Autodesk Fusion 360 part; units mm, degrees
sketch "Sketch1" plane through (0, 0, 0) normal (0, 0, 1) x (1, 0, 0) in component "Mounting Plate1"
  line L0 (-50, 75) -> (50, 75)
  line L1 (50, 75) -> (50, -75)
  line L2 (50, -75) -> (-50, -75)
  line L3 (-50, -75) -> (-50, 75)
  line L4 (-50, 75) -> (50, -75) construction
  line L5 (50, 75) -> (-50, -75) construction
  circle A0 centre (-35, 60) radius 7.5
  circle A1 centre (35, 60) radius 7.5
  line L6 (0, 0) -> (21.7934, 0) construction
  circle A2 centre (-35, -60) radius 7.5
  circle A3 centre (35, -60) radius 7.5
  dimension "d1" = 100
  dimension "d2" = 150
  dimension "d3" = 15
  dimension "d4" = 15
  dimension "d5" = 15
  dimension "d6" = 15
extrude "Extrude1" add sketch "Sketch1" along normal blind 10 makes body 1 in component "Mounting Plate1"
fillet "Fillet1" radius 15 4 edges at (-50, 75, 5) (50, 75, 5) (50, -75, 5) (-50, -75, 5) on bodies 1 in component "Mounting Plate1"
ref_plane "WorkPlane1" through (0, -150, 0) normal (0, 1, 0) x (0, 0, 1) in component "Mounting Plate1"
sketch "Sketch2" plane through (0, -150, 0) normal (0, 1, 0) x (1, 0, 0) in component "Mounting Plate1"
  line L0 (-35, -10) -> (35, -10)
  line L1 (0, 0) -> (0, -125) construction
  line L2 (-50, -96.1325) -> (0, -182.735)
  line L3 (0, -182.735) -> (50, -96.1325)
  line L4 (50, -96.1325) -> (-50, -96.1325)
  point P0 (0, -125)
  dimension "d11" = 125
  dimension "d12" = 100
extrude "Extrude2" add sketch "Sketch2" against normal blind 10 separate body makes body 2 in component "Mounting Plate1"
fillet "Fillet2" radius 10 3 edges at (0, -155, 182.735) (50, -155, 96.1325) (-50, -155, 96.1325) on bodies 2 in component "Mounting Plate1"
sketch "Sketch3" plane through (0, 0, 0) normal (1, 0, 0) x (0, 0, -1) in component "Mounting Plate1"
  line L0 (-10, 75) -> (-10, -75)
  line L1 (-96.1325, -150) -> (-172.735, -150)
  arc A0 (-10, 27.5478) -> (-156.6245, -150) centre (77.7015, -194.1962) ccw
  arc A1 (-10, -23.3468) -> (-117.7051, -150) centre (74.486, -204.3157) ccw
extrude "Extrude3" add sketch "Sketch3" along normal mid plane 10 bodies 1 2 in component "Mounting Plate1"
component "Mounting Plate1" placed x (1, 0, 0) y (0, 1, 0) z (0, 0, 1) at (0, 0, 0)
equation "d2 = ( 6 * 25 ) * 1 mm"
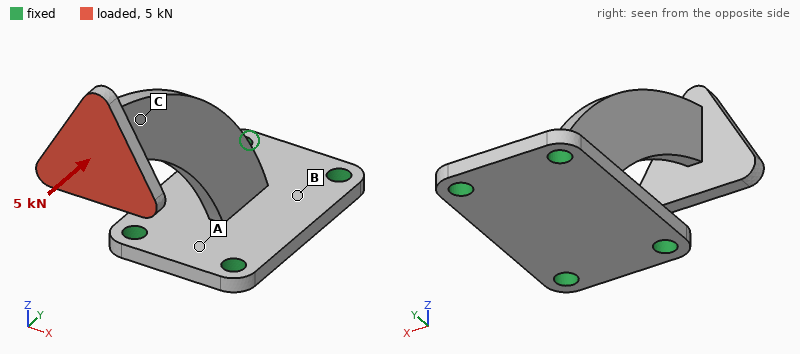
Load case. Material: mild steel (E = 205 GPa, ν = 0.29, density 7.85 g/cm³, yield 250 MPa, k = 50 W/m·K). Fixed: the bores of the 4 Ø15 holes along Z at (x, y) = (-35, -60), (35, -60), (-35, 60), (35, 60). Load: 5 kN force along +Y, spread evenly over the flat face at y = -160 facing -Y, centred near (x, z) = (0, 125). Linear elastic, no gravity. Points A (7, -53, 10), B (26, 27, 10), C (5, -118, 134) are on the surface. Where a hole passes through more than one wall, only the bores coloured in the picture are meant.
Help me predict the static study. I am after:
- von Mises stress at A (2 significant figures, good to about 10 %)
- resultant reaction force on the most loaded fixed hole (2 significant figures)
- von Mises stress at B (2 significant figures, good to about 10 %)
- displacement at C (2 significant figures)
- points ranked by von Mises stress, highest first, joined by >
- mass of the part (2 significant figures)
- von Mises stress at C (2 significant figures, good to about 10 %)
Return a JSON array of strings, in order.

["35 MPa", "3.9 kN", "49 MPa", "0.61 mm", "B > A > C", "2.1 kg", "14 MPa"]
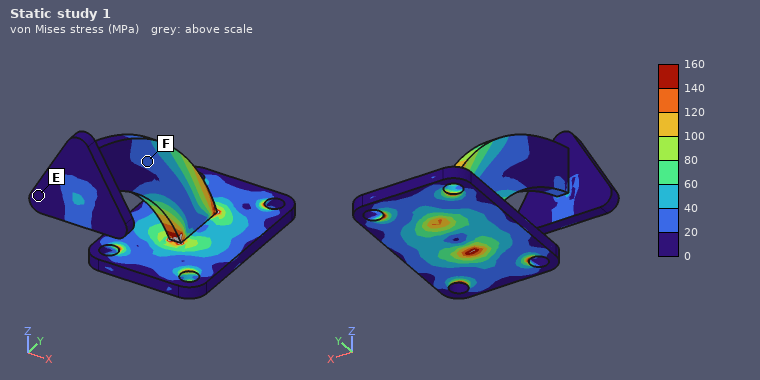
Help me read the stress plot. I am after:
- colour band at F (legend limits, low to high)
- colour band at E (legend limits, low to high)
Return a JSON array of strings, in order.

["20 to 40 MPa", "0 to 20 MPa"]
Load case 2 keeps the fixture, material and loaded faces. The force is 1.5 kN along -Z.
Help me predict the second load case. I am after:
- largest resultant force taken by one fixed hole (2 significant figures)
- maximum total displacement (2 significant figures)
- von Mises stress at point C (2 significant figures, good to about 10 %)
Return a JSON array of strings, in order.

["1.8 kN", "0.46 mm", "10 MPa"]
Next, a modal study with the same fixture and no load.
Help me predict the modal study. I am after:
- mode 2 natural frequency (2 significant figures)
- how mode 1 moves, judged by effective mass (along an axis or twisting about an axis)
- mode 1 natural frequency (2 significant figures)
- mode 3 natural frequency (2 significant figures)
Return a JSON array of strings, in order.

["420 Hz", "along X", "130 Hz", "570 Hz"]
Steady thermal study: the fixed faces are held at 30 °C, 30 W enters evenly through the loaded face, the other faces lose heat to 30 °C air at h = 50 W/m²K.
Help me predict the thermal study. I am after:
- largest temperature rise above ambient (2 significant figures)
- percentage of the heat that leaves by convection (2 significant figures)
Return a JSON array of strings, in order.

["53 K", "98 %"]
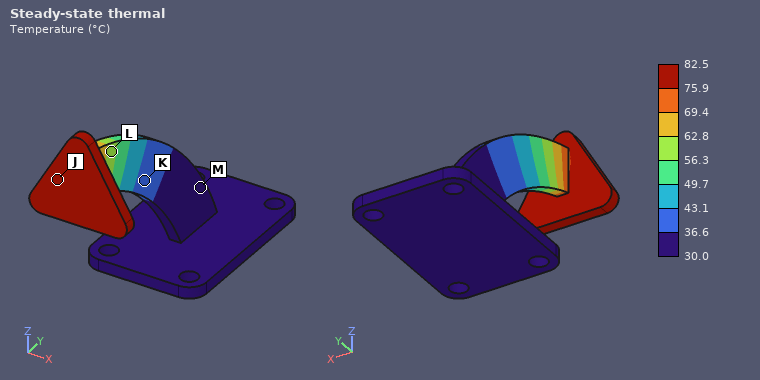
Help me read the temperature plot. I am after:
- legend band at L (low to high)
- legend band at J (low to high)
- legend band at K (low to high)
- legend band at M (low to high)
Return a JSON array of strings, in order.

["56.3 to 62.8 °C", "75.9 to 82.5 °C", "36.6 to 43.1 °C", "30.0 to 36.6 °C"]
